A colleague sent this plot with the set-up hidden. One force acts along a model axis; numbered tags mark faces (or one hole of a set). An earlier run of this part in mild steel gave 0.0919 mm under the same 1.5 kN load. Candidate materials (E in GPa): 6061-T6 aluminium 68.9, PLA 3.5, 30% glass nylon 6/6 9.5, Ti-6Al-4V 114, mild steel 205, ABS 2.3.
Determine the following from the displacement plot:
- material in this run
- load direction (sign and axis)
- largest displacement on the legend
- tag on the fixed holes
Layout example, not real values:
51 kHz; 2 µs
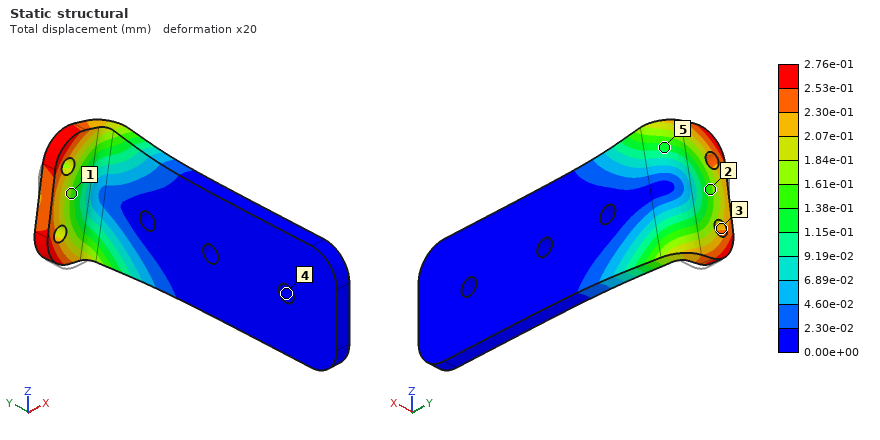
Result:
6061-T6 aluminium; +Z; 2.76e-01 mm; 4
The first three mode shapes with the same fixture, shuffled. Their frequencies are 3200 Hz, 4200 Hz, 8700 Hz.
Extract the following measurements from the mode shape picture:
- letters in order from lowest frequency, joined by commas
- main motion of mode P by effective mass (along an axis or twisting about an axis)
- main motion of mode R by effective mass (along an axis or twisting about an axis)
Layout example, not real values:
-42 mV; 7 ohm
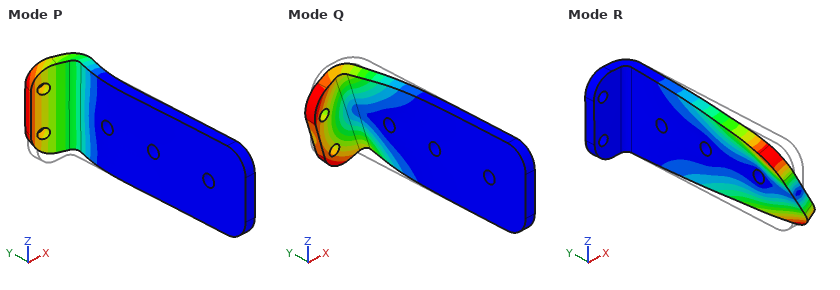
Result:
P, Q, R; along X; twisting about Y
